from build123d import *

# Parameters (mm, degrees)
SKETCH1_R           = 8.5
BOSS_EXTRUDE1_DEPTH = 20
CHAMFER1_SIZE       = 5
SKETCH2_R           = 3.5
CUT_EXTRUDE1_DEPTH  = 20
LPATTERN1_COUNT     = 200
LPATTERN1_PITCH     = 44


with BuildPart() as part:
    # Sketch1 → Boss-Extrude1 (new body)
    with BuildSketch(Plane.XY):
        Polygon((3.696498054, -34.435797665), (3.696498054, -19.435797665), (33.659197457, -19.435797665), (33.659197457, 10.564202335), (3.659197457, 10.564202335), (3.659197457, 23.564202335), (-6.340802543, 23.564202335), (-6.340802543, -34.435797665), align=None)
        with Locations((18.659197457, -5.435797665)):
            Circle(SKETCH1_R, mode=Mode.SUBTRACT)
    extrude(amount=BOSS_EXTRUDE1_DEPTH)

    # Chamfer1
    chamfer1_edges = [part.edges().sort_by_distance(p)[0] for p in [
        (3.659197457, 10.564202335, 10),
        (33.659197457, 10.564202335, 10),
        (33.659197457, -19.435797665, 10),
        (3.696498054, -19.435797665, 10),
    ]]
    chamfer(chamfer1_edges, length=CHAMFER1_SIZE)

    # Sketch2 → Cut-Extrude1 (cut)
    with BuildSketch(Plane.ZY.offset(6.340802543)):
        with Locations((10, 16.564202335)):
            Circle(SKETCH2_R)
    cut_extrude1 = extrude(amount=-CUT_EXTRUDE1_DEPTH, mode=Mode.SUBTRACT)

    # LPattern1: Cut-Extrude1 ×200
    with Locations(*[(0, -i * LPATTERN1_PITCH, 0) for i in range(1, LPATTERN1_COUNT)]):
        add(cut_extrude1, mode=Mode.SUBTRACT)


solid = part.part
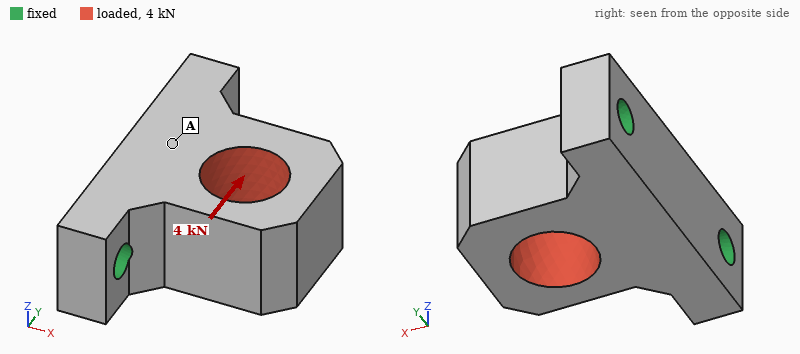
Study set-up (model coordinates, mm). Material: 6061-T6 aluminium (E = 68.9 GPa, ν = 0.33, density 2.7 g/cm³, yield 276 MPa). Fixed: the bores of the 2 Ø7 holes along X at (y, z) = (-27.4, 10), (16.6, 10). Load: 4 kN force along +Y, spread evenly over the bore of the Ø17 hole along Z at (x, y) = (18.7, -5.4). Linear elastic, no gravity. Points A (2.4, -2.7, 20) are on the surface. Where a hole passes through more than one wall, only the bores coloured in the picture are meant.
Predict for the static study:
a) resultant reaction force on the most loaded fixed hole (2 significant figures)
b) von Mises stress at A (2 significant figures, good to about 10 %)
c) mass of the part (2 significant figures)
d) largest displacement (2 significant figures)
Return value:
2.8 kN
8.2 MPa
66 g
26 µm
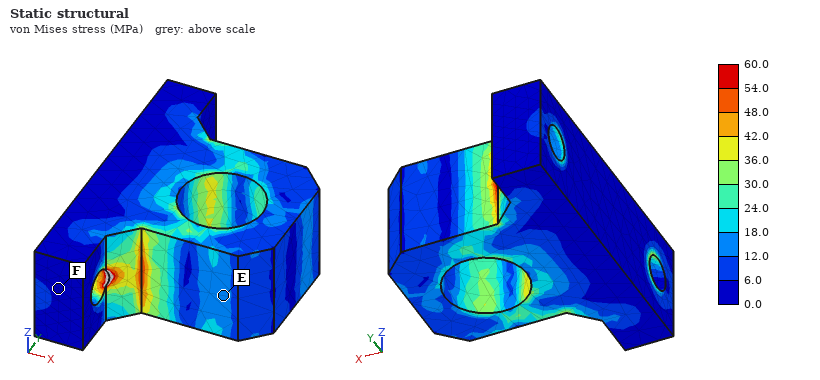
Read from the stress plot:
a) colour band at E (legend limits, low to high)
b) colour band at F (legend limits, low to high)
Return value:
12.0 to 18.0 MPa
0.0 to 6.0 MPa
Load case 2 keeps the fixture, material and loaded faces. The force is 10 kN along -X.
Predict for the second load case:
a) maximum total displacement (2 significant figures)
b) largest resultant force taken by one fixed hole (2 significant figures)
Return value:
22 µm
5.4 kN
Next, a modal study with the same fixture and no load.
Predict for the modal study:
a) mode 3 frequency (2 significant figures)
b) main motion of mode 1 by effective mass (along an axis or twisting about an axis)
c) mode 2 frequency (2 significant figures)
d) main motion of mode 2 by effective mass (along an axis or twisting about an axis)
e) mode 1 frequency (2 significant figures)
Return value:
17 kHz
along Z
12 kHz
along Y
6900 Hz
